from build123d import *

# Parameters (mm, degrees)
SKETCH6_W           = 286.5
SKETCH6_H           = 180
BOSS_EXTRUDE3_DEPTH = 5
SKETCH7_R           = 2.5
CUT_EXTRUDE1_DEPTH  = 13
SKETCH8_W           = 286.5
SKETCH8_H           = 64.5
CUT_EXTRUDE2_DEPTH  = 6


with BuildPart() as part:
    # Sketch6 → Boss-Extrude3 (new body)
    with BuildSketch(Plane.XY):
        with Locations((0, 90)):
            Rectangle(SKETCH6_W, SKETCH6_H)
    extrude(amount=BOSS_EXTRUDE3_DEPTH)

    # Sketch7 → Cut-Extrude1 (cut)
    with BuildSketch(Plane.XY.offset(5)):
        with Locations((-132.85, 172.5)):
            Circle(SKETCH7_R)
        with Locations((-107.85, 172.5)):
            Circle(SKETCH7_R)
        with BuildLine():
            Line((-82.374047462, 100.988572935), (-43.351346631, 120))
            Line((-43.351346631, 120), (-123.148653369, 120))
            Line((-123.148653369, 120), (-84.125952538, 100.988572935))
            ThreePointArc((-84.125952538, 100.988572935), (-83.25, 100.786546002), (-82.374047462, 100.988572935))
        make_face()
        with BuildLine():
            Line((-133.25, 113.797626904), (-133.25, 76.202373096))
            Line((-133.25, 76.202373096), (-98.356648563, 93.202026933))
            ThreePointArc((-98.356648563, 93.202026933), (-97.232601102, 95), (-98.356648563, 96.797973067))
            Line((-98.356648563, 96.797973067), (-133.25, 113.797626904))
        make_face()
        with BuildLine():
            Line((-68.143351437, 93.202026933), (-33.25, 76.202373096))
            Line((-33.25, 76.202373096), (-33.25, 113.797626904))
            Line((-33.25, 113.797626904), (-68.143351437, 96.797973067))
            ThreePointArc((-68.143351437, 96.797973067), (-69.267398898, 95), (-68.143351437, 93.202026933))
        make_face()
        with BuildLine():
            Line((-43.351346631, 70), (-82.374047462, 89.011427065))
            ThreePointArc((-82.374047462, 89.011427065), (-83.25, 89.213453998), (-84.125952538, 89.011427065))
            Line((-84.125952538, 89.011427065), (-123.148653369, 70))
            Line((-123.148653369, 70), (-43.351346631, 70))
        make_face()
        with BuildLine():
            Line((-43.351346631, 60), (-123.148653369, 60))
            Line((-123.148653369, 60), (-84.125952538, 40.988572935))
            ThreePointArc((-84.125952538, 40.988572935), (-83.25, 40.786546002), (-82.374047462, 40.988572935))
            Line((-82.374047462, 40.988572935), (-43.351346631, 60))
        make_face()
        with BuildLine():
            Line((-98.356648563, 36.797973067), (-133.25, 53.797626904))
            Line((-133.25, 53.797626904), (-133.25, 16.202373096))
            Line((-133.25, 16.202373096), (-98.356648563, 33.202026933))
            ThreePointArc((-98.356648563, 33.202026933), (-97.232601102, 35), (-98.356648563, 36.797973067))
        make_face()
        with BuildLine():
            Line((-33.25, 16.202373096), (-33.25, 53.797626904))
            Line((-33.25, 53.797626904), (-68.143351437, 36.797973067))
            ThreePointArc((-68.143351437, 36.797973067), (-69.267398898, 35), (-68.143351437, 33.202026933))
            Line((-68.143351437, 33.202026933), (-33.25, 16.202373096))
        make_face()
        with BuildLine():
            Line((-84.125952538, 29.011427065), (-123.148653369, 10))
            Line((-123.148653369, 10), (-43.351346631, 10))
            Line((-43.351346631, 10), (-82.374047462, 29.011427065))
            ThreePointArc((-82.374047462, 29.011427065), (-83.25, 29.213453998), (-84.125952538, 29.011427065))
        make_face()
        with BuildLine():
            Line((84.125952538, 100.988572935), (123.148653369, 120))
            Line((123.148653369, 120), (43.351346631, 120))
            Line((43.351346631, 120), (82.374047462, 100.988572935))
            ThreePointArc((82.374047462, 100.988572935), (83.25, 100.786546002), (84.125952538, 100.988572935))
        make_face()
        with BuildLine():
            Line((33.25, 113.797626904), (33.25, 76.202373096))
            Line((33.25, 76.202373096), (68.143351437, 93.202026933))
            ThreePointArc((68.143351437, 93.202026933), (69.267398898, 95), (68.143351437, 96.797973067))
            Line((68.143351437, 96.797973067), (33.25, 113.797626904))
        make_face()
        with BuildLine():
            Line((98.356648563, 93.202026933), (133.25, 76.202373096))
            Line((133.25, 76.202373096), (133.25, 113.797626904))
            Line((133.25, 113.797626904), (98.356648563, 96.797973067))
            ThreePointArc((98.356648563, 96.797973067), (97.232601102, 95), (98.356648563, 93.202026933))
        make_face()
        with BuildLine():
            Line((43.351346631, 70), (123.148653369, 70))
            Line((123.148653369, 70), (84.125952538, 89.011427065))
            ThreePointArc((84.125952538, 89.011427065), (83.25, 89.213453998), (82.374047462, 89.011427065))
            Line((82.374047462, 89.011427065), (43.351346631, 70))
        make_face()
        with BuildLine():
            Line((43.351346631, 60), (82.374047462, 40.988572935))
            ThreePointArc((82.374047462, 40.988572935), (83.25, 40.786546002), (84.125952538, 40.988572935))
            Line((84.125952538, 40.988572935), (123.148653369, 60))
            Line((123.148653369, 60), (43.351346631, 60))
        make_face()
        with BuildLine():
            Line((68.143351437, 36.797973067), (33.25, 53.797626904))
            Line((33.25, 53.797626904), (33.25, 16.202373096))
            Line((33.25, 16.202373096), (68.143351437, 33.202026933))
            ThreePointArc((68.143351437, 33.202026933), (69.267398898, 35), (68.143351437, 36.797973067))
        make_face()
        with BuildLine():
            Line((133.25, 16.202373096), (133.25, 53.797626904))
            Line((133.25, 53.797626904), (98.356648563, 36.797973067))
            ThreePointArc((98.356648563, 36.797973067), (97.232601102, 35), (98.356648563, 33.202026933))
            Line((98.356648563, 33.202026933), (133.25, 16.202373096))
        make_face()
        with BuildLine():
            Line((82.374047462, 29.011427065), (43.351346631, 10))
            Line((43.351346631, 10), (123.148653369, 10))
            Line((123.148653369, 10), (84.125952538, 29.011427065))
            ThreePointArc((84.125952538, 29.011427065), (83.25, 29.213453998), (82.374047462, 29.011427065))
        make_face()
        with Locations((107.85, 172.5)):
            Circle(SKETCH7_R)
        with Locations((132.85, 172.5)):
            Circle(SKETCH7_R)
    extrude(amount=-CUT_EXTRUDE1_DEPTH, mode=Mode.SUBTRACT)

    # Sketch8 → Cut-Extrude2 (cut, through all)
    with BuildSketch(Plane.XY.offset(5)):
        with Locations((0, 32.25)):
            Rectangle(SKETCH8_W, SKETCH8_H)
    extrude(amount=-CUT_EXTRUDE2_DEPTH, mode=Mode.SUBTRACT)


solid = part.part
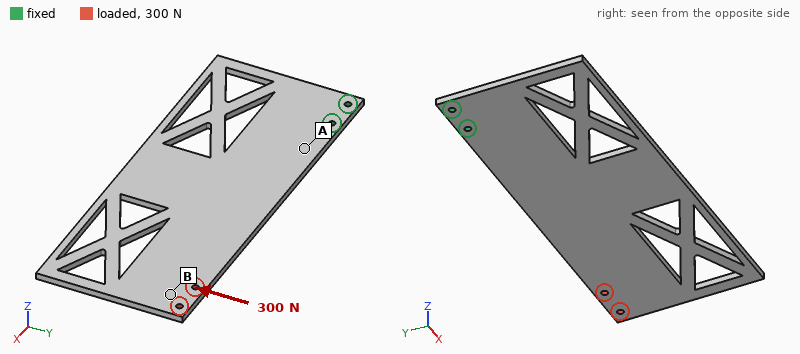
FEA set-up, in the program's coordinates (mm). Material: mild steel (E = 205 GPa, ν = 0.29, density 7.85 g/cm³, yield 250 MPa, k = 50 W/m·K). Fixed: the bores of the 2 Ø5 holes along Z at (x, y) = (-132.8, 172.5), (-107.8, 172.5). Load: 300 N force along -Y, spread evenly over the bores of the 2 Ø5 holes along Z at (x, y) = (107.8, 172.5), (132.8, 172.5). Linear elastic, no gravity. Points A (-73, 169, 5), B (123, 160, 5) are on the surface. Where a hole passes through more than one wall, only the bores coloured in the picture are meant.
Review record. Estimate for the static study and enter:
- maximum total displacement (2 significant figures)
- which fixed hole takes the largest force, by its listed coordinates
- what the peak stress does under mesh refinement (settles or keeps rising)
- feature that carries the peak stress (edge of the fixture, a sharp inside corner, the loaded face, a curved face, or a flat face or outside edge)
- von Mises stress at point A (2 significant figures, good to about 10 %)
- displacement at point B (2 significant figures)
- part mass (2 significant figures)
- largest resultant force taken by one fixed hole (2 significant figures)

0.11 mm
(-107.8, 172.5)
keeps rising
edge of the fixture
8.4 MPa
0.092 mm
1.1 kg
2.7 kN
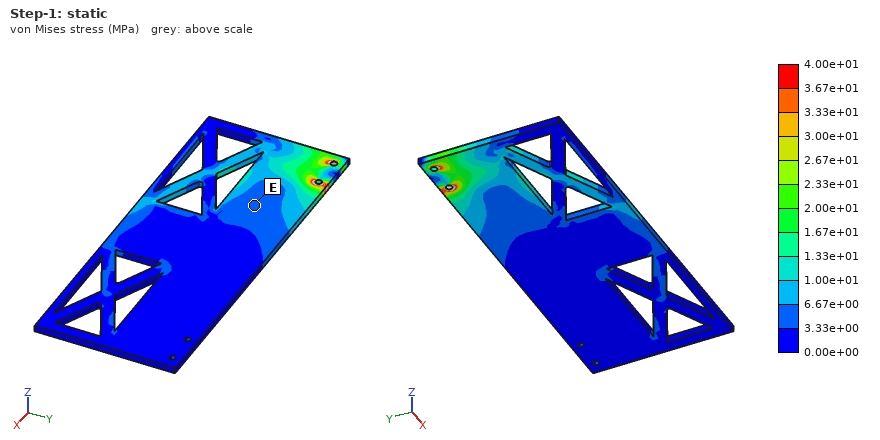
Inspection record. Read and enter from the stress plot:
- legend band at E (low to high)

3.33e+00 to 6.67e+00 MPa
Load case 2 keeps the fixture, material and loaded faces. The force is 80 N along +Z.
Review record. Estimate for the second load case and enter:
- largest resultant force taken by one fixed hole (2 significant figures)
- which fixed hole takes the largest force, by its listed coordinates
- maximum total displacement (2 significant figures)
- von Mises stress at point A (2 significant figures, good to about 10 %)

470 N
(-107.8, 172.5)
2.5 mm
52 MPa
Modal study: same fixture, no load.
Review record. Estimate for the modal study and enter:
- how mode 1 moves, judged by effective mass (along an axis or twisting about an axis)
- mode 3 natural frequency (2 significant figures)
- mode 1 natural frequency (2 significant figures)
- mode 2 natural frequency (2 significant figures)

along Z
350 Hz
54 Hz
200 Hz
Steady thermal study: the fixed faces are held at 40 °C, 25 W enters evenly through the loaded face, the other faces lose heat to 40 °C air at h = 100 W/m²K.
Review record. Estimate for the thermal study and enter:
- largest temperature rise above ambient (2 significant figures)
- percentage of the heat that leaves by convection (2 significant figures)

58 K
100 %
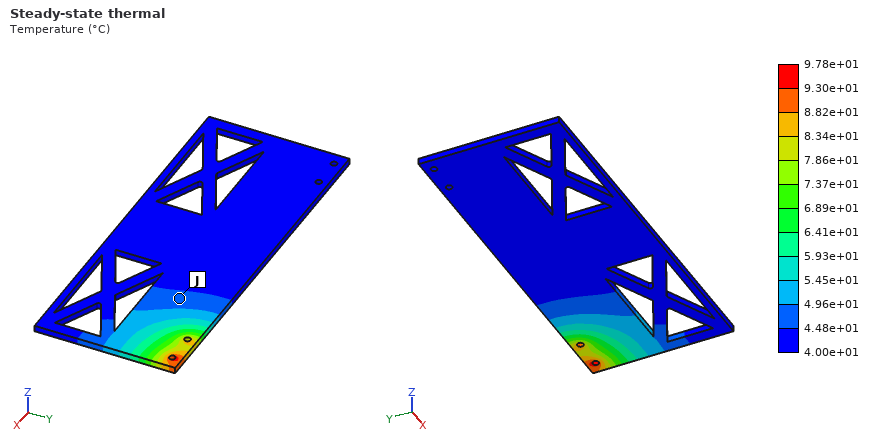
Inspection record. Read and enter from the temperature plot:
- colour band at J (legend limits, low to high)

4.48e+01 to 4.96e+01 °C
